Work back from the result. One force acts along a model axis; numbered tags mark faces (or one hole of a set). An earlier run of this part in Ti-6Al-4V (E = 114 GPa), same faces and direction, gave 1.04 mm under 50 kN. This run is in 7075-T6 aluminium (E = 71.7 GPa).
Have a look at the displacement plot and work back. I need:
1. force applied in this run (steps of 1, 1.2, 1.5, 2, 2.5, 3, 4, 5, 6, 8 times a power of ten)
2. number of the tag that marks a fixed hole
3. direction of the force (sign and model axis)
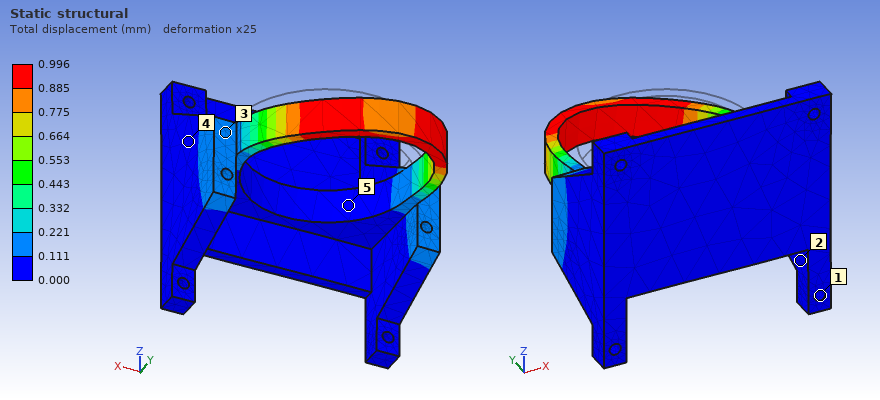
30 kN
1
-X
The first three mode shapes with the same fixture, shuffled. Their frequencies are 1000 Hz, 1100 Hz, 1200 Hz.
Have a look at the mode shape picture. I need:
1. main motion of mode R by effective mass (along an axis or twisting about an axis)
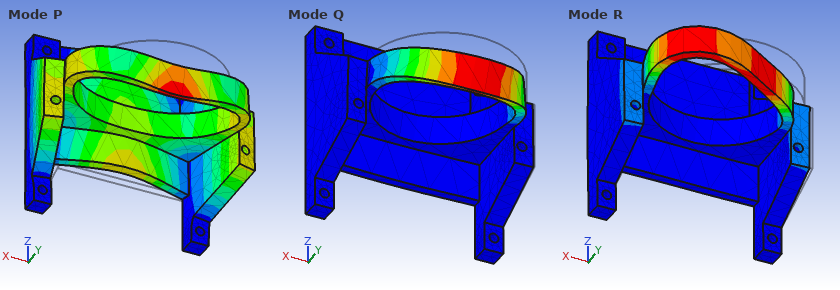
along X
